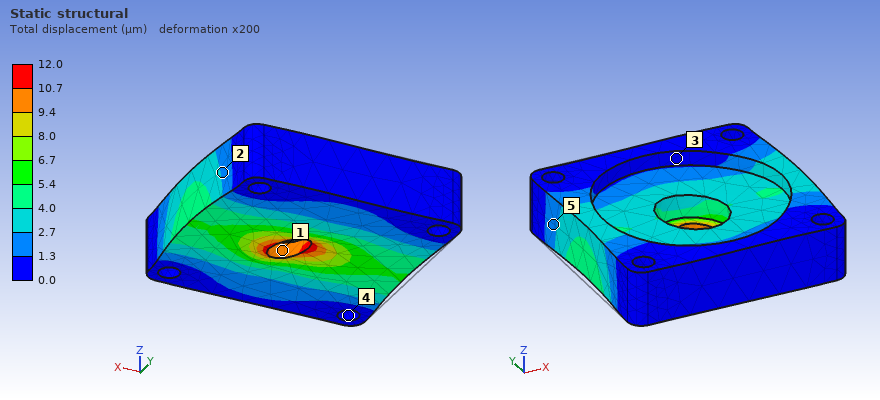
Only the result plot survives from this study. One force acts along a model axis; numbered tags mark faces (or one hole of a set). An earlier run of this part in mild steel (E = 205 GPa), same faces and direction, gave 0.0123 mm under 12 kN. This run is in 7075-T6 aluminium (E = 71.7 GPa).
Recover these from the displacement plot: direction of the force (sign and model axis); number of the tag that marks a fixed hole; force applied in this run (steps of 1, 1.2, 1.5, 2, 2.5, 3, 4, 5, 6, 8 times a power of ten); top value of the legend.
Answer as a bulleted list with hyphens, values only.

- +X
- 4
- 4 kN
- 12.0 µm
